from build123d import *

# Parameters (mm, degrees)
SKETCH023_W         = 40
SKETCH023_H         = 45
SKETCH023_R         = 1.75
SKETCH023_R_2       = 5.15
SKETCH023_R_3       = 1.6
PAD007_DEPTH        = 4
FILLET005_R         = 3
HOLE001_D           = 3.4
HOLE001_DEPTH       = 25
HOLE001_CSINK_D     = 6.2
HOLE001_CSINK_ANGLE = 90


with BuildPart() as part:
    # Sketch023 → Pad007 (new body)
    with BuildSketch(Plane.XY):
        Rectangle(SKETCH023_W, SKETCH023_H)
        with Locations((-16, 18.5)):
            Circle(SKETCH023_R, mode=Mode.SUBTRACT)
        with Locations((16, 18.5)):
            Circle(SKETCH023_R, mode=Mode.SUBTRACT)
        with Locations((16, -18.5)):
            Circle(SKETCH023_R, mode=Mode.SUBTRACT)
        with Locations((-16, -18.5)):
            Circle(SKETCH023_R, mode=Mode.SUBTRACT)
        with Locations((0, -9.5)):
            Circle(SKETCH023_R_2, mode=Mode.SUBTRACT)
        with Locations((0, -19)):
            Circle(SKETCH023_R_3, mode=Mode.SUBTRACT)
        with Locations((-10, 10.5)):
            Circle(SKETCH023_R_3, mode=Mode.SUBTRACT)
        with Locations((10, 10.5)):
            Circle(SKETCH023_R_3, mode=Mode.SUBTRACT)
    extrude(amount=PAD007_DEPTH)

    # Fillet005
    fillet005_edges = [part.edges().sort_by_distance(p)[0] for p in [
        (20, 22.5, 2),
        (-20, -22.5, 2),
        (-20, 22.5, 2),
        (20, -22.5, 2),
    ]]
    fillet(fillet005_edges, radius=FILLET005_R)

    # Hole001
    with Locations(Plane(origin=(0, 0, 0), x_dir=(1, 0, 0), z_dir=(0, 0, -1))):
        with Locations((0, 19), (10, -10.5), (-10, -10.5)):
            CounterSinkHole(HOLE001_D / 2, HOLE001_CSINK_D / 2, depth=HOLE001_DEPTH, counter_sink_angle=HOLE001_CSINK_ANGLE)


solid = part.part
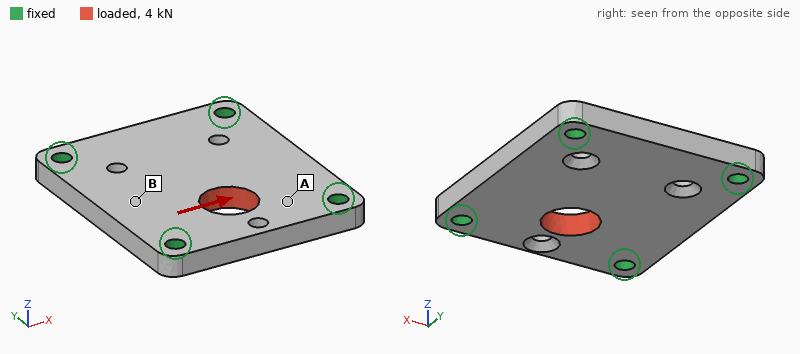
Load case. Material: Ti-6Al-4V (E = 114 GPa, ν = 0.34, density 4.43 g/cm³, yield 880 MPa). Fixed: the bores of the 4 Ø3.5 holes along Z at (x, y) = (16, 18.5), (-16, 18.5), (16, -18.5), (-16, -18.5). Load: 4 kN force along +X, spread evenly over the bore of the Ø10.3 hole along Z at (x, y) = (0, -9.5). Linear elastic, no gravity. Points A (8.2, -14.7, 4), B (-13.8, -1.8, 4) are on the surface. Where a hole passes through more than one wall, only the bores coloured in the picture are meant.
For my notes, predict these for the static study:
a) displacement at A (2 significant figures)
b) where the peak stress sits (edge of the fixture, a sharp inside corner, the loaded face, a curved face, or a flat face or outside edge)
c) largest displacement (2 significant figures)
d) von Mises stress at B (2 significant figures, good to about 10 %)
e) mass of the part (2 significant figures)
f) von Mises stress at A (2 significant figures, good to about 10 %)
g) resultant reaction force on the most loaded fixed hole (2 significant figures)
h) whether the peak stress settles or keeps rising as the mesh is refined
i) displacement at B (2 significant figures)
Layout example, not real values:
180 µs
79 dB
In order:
3.3 µm
edge of the fixture
7.4 µm
13 MPa
29 g
34 MPa
1.5 kN
keeps rising
5.3 µm
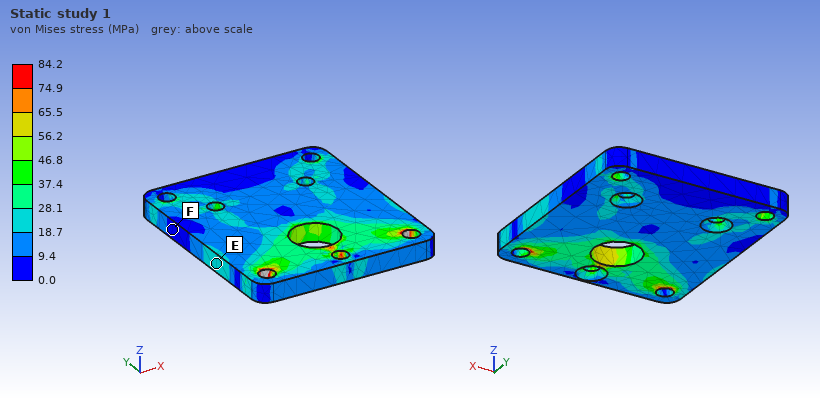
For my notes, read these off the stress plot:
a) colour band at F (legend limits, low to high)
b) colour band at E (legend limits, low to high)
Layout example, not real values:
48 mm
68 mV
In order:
0.0 to 9.4 MPa
18.7 to 28.1 MPa
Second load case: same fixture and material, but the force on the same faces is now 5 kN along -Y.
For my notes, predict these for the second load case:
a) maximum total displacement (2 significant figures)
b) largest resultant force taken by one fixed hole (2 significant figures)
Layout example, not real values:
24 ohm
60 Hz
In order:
13 µm
1.6 kN
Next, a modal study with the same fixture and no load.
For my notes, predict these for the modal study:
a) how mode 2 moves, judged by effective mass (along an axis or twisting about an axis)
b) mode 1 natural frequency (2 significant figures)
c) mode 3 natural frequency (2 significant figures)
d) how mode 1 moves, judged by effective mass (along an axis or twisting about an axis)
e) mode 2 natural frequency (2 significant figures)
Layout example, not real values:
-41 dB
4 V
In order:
twisting about Y
11 kHz
20 kHz
along Z
17 kHz
